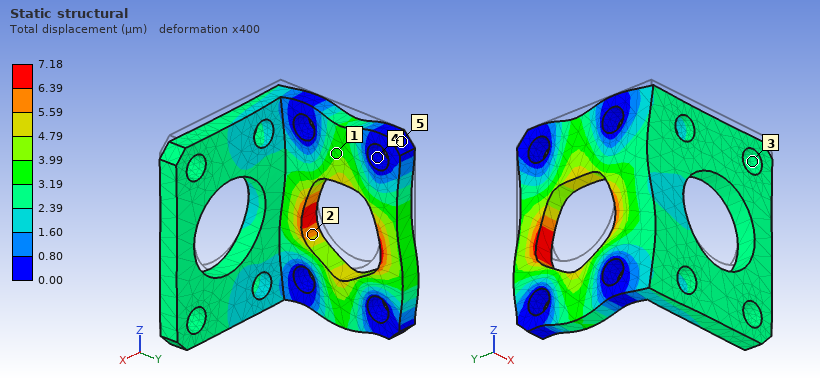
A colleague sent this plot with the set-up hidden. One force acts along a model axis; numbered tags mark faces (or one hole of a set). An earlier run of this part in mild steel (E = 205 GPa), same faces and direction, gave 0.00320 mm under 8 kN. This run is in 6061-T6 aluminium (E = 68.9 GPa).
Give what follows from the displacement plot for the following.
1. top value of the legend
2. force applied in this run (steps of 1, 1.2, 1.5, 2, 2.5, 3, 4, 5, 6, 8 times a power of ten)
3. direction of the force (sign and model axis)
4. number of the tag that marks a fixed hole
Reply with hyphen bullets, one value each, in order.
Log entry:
- 7.18 µm
- 6 kN
- -Z
- 4
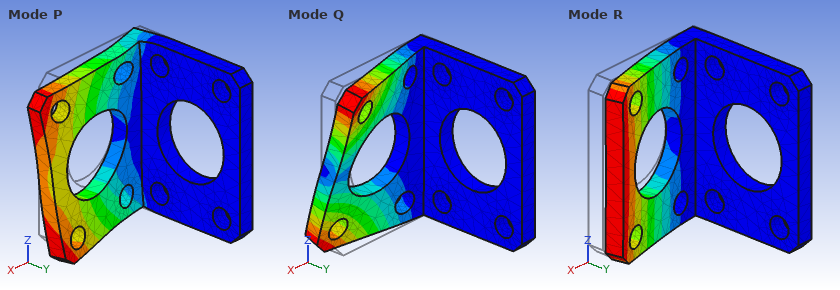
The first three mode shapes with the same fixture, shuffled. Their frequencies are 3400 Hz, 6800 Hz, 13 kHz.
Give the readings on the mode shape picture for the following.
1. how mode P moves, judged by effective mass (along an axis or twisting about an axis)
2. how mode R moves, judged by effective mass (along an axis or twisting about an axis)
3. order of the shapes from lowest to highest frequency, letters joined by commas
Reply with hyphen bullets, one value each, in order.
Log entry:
- along Z
- along Y
- R, Q, P
